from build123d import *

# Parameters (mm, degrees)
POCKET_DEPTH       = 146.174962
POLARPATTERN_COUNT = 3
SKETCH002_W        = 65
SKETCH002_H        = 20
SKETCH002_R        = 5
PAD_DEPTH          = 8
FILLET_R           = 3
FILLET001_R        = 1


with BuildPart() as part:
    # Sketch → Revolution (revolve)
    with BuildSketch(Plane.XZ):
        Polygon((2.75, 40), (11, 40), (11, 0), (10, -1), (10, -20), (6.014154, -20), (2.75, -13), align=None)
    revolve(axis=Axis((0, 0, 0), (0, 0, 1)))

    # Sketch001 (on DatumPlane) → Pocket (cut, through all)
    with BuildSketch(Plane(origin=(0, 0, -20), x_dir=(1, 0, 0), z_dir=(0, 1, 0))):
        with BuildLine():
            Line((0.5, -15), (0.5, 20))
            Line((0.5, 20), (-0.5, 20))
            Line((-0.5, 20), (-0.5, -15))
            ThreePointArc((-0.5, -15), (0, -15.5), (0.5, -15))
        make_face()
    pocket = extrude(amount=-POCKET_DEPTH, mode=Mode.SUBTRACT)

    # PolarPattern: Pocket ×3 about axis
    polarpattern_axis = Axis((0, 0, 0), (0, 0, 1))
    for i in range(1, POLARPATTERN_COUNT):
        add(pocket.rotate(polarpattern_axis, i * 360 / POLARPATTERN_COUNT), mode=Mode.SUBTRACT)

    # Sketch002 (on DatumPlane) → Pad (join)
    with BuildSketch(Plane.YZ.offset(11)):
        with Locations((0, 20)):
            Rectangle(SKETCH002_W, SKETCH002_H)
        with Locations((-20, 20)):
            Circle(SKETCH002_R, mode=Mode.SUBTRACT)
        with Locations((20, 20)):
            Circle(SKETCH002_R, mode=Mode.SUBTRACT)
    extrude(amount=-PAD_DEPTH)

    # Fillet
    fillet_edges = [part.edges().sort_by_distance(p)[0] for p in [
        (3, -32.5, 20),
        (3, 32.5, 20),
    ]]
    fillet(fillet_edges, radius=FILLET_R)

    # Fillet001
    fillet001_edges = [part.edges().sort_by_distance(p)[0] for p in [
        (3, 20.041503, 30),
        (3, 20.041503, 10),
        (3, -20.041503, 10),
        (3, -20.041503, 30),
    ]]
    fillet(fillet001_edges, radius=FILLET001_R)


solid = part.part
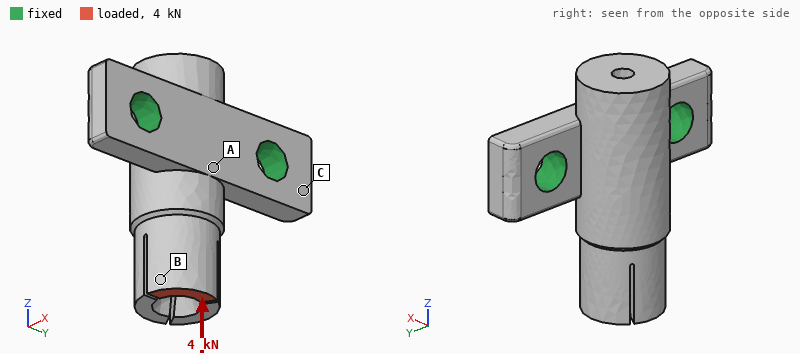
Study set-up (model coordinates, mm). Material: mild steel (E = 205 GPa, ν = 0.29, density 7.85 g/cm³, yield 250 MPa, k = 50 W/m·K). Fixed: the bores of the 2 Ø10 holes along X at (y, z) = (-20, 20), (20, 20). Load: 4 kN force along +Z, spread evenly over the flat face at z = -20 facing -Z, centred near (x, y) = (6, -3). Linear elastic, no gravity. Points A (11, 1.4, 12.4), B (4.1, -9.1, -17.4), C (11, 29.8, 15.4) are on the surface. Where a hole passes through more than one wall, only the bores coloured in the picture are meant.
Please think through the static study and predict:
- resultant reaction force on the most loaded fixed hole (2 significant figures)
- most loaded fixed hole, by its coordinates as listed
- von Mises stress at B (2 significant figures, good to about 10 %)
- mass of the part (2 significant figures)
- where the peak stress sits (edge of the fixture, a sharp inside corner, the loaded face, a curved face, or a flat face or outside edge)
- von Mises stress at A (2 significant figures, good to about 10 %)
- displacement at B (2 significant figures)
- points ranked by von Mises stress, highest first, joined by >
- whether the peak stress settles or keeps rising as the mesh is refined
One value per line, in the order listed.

2.4 kN
(-20, 20)
71 MPa
200 g
a sharp inside corner
19 MPa
16 µm
B > A > C
keeps rising
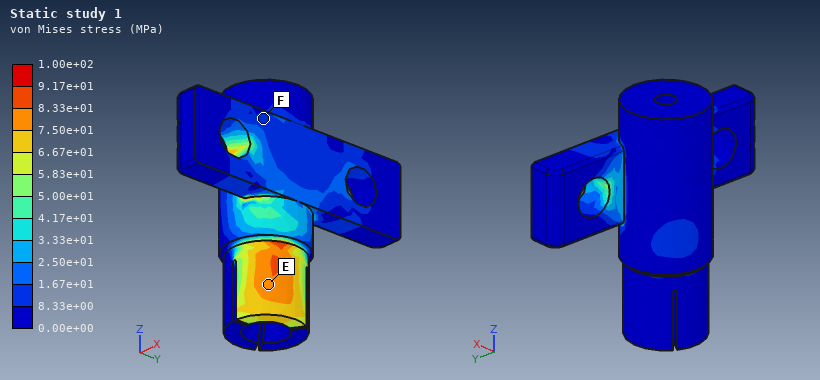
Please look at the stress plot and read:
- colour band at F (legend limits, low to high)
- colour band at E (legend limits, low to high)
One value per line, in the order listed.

8.33e+00 to 1.67e+01 MPa
7.50e+01 to 8.33e+01 MPa
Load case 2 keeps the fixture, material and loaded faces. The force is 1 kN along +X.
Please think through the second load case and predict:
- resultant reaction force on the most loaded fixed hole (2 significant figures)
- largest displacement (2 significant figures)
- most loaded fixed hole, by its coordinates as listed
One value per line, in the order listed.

740 N
67 µm
(-20, 20)
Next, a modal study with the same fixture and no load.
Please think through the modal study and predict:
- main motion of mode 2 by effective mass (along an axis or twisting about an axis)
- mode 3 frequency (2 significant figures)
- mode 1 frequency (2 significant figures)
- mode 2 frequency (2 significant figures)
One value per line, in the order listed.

along Y
14 kHz
4600 Hz
9300 Hz
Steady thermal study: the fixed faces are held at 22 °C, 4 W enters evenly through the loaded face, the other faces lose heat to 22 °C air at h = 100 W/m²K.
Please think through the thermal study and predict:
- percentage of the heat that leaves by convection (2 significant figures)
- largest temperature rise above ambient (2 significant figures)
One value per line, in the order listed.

49 %
20 K
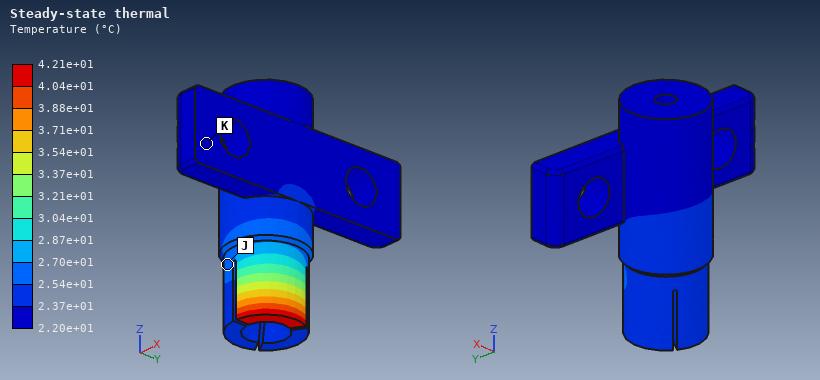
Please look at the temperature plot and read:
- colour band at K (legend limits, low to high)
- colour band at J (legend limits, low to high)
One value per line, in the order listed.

2.20e+01 to 2.37e+01 °C
2.54e+01 to 2.70e+01 °C
